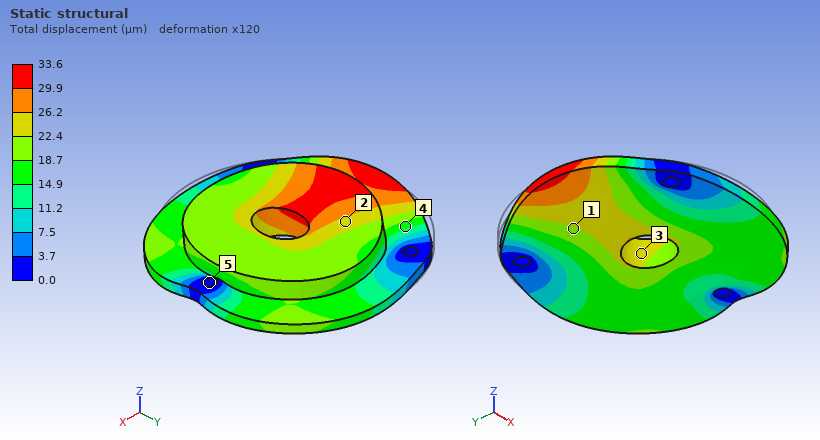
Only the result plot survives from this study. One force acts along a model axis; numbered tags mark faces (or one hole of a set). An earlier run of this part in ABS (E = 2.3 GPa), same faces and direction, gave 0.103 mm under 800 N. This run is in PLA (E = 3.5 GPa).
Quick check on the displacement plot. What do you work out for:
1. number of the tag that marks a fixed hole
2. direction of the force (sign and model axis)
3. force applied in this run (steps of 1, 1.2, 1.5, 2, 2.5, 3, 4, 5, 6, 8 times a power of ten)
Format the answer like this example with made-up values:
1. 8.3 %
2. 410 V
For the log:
1. 5
2. +X
3. 400 N
